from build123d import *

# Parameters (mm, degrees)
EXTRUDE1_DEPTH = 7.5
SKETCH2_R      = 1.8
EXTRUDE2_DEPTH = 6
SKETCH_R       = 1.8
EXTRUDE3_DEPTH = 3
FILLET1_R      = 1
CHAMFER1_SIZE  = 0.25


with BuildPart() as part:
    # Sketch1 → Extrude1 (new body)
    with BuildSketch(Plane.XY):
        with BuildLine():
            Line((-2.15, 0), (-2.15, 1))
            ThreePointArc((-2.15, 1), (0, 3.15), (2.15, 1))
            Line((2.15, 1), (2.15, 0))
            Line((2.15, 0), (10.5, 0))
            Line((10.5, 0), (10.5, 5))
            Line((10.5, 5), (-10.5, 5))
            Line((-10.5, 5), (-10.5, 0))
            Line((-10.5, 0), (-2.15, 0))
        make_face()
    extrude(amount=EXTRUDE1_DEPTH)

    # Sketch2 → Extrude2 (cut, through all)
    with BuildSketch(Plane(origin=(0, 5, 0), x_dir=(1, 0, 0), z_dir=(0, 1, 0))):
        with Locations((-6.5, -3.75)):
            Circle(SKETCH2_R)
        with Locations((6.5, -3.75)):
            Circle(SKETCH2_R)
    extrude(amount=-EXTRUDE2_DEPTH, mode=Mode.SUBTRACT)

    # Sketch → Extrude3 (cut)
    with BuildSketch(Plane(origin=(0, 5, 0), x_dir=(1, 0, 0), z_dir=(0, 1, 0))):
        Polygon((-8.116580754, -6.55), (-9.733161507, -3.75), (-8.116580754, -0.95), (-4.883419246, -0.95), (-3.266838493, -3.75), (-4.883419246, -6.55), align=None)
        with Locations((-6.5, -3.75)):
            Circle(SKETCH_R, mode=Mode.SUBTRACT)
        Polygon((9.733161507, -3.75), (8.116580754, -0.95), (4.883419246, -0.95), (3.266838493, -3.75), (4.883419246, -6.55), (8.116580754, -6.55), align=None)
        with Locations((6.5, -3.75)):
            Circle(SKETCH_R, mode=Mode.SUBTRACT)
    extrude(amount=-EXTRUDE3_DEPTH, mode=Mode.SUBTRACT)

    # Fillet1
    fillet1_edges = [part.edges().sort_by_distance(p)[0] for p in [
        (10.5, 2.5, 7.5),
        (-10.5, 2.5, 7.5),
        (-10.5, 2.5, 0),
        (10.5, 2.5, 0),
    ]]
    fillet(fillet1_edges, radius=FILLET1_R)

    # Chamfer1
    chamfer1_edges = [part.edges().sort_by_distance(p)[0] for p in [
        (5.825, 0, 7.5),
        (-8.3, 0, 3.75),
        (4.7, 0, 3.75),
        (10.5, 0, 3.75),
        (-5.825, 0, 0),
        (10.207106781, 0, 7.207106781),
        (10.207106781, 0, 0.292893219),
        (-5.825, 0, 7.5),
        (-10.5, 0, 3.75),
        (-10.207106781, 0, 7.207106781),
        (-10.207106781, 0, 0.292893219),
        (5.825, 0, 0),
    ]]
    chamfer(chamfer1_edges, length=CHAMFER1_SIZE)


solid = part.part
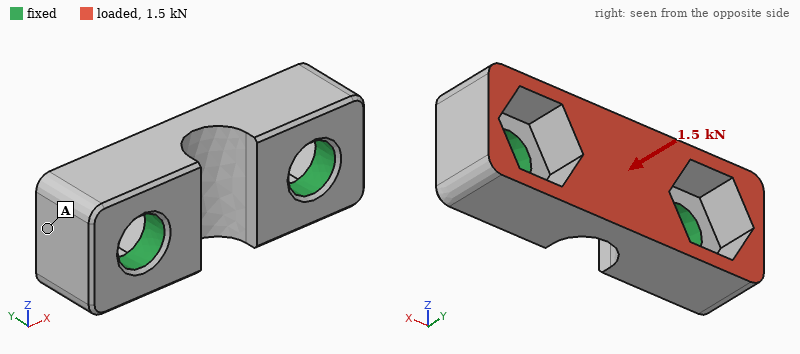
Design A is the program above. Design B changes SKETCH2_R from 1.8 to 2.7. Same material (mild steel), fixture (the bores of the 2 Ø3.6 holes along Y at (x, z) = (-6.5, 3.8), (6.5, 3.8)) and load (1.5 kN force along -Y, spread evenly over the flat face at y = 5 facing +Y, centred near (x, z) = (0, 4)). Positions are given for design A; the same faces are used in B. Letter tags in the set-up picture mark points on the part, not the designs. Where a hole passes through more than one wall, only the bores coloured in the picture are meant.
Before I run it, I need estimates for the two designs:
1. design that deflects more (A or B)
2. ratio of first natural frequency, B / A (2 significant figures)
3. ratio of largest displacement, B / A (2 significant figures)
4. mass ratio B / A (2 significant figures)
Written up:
A
1.5
0.58
0.90
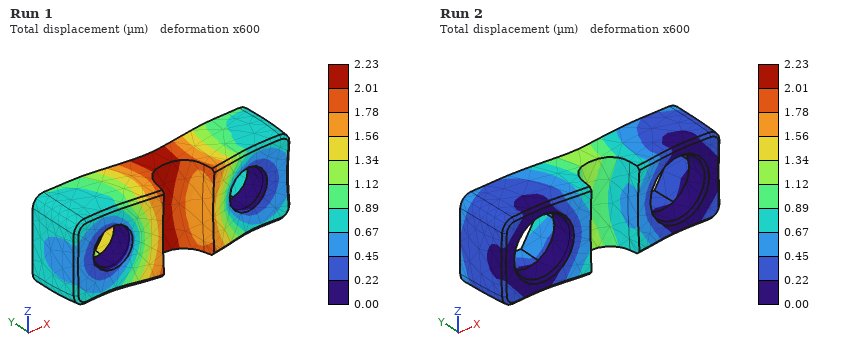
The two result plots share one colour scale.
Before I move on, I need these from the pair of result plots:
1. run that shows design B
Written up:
Run 2
